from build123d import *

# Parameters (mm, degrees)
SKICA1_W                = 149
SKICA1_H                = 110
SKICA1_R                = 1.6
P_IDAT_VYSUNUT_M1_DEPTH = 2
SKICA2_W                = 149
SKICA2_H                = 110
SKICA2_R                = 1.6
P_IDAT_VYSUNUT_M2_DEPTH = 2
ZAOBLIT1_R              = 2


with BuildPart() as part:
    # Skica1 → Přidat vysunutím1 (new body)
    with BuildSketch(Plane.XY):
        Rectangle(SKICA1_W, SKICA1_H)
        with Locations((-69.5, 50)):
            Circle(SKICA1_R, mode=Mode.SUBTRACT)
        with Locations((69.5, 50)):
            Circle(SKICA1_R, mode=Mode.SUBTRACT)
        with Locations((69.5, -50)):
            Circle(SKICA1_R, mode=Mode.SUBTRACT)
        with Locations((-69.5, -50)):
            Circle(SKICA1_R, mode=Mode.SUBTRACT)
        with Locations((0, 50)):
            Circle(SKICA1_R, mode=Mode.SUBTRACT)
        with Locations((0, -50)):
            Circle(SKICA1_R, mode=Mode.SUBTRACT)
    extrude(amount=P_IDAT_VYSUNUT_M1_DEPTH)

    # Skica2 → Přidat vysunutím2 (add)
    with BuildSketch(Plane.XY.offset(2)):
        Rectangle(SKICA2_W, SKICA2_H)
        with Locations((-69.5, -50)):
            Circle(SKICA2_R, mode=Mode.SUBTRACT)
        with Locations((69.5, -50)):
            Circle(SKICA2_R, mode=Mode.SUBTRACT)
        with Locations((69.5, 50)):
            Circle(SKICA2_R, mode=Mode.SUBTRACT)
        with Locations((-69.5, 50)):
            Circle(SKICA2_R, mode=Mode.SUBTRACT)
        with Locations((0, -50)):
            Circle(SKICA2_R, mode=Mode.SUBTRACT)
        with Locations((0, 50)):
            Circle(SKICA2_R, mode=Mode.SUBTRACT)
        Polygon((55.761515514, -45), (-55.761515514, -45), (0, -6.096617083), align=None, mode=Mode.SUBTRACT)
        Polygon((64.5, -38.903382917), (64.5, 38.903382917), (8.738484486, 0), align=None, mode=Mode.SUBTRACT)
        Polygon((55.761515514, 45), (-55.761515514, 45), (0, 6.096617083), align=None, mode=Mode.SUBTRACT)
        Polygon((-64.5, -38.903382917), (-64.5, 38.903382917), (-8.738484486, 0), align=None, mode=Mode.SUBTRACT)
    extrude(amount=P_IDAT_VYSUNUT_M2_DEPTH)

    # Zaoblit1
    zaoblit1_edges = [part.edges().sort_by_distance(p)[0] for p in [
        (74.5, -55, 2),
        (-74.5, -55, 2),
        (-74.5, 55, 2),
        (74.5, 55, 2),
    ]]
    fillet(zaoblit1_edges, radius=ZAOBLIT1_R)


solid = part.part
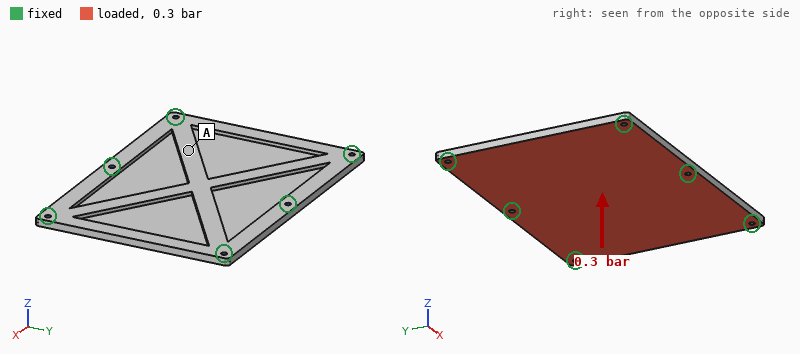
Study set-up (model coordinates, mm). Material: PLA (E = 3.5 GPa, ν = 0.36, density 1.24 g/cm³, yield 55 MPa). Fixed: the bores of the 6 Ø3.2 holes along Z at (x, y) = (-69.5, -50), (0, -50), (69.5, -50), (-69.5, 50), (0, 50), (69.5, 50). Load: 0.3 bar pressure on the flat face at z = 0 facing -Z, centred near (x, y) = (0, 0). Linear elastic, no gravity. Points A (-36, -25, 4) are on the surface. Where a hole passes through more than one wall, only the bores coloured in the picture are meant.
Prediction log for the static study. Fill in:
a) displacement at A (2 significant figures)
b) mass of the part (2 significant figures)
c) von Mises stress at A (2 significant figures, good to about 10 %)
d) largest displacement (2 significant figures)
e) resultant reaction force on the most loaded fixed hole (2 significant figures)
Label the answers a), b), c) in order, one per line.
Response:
a) 1.1 mm
b) 60 g
c) 3.3 MPa
d) 1.8 mm
e) 140 N
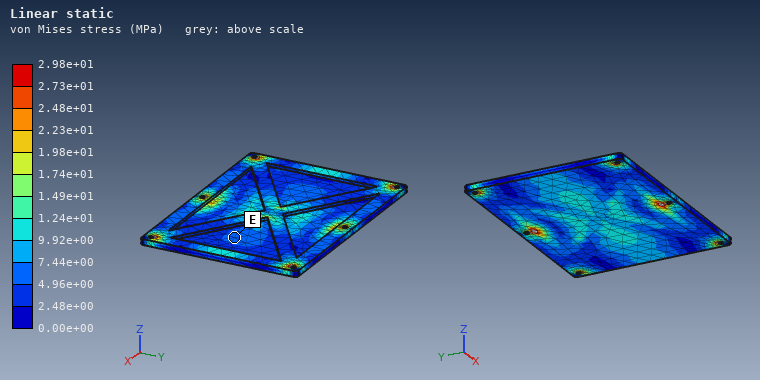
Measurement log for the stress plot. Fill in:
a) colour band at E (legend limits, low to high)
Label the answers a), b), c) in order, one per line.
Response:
a) 4.96e+00 to 7.44e+00 MPa
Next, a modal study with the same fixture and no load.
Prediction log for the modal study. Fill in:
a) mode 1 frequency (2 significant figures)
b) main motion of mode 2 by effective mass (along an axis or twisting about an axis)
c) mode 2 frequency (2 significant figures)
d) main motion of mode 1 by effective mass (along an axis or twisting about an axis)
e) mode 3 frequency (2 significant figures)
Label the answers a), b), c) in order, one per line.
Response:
a) 430 Hz
b) twisting about Y
c) 580 Hz
d) along Z
e) 790 Hz
